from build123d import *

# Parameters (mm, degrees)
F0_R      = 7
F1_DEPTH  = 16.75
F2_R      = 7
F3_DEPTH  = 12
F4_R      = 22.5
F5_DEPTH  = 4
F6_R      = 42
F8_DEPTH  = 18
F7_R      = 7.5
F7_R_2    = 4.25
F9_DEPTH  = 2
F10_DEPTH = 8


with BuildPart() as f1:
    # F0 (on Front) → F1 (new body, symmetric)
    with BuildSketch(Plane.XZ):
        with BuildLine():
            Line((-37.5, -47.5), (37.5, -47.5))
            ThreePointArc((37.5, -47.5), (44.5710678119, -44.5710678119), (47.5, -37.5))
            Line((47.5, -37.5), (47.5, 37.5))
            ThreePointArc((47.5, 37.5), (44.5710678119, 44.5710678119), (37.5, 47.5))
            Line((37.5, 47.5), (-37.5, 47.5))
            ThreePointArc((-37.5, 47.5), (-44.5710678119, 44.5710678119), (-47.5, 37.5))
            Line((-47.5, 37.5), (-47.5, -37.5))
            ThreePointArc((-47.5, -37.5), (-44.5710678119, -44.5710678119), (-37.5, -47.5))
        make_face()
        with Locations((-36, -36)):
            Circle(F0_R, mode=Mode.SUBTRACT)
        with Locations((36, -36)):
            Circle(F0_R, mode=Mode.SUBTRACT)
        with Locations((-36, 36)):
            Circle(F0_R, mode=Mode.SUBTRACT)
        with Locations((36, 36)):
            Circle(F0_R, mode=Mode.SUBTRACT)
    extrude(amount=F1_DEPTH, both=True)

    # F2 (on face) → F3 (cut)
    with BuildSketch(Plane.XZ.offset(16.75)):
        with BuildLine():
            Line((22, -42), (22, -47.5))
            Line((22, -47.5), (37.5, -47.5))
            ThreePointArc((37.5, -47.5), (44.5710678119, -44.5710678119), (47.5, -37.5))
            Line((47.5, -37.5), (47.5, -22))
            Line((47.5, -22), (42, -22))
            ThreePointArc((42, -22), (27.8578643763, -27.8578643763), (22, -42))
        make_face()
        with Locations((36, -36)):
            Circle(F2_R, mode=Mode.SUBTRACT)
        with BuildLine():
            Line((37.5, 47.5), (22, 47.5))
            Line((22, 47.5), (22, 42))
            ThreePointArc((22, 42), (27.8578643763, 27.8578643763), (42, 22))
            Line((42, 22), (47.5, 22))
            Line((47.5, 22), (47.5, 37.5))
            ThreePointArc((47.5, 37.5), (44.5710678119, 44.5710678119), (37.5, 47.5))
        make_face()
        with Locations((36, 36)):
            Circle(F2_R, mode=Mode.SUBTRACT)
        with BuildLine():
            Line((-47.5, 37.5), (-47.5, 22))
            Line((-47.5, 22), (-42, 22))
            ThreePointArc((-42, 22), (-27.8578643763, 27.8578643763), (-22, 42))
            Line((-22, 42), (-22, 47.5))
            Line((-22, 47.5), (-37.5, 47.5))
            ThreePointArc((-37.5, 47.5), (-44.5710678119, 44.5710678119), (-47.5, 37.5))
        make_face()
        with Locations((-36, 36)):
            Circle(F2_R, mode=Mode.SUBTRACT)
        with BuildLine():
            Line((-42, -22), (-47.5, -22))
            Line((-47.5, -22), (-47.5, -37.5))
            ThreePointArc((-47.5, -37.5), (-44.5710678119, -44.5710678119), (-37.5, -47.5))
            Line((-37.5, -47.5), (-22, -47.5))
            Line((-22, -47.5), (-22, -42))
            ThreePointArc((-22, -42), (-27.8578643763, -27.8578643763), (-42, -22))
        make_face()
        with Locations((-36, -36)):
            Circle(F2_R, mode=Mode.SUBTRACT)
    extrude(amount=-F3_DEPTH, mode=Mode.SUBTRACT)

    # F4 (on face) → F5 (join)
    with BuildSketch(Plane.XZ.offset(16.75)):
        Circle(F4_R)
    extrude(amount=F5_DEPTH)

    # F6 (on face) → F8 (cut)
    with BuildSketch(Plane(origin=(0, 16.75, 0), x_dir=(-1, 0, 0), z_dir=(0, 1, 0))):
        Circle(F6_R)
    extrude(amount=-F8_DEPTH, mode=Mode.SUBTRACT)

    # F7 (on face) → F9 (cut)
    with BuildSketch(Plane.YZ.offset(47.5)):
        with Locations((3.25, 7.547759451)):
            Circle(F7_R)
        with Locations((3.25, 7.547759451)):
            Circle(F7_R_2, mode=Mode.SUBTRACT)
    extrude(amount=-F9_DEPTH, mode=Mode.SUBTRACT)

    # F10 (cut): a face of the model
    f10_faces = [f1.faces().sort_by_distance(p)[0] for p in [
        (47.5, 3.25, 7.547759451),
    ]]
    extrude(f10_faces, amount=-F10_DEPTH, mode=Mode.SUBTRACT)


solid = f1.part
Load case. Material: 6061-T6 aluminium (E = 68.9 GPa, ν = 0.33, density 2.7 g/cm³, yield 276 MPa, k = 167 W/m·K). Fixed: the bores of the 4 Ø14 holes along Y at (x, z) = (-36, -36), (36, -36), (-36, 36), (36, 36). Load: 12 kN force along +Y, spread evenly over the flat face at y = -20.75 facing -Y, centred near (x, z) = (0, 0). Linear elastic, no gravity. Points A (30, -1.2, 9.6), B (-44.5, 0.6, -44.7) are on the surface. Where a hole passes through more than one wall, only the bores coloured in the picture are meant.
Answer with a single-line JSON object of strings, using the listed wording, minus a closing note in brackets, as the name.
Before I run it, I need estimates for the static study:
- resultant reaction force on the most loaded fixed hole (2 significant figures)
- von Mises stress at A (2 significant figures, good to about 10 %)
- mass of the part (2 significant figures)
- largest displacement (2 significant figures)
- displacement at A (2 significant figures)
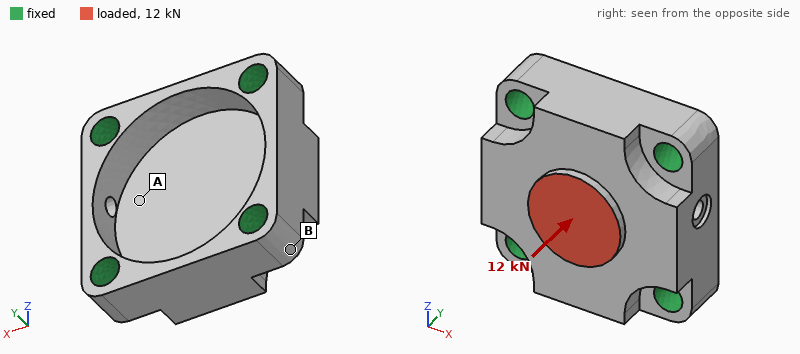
{"resultant reaction force on the most loaded fixed hole": "4.1 kN", "von Mises stress at A": "8.0 MPa", "mass of the part": "450 g", "largest displacement": "23 µm", "displacement at A": "11 µm"}
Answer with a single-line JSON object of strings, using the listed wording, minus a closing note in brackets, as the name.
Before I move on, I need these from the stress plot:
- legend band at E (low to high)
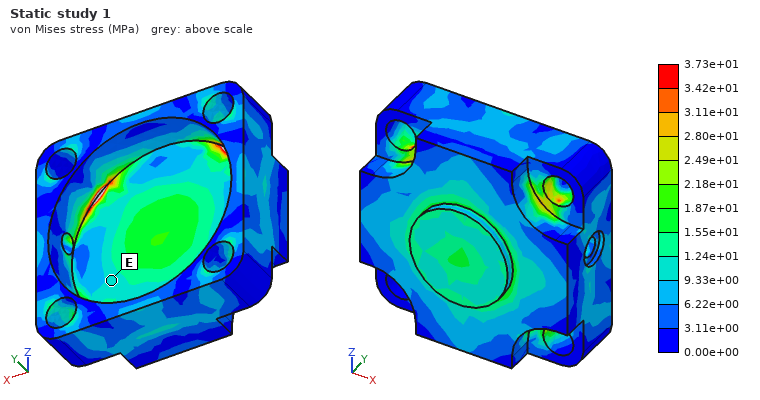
{"legend band at E": "9.33e+00 to 1.24e+01 MPa"}
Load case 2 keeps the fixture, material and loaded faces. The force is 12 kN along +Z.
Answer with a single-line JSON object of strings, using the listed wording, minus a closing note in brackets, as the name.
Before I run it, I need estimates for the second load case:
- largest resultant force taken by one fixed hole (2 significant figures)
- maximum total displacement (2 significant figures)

{"largest resultant force taken by one fixed hole": "3.7 kN", "maximum total displacement": "12 µm"}
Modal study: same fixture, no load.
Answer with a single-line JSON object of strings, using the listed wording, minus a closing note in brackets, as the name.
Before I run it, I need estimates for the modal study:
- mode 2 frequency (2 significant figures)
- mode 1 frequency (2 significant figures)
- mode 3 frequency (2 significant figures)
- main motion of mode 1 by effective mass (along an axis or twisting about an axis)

{"mode 2 frequency": "14 kHz", "mode 1 frequency": "10 kHz", "mode 3 frequency": "14 kHz", "main motion of mode 1 by effective mass": "along Y"}
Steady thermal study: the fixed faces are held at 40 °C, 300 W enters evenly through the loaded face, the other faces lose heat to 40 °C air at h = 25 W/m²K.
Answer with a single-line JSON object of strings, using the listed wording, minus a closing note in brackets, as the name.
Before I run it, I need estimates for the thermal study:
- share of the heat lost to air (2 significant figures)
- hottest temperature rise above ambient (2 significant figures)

{"share of the heat lost to air": "3.1 %", "hottest temperature rise above ambient": "42 K"}
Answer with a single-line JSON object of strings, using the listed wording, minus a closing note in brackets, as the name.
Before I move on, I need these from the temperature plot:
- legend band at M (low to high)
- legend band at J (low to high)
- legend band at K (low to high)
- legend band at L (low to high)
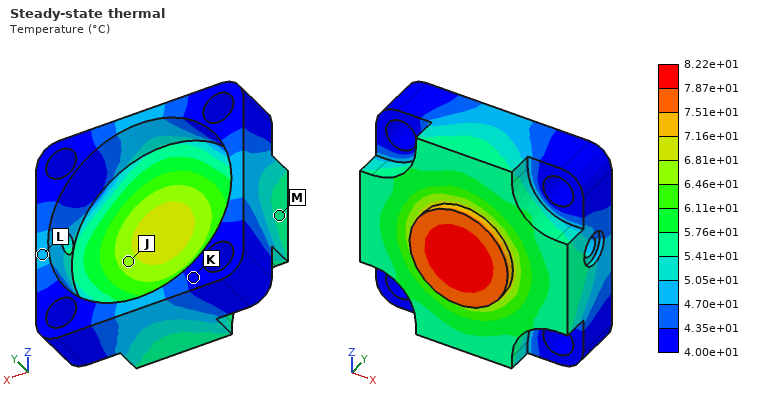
{"legend band at M": "5.41e+01 to 5.76e+01 °C", "legend band at J": "6.46e+01 to 6.81e+01 °C", "legend band at K": "4.00e+01 to 4.35e+01 °C", "legend band at L": "4.70e+01 to 5.05e+01 °C"}
